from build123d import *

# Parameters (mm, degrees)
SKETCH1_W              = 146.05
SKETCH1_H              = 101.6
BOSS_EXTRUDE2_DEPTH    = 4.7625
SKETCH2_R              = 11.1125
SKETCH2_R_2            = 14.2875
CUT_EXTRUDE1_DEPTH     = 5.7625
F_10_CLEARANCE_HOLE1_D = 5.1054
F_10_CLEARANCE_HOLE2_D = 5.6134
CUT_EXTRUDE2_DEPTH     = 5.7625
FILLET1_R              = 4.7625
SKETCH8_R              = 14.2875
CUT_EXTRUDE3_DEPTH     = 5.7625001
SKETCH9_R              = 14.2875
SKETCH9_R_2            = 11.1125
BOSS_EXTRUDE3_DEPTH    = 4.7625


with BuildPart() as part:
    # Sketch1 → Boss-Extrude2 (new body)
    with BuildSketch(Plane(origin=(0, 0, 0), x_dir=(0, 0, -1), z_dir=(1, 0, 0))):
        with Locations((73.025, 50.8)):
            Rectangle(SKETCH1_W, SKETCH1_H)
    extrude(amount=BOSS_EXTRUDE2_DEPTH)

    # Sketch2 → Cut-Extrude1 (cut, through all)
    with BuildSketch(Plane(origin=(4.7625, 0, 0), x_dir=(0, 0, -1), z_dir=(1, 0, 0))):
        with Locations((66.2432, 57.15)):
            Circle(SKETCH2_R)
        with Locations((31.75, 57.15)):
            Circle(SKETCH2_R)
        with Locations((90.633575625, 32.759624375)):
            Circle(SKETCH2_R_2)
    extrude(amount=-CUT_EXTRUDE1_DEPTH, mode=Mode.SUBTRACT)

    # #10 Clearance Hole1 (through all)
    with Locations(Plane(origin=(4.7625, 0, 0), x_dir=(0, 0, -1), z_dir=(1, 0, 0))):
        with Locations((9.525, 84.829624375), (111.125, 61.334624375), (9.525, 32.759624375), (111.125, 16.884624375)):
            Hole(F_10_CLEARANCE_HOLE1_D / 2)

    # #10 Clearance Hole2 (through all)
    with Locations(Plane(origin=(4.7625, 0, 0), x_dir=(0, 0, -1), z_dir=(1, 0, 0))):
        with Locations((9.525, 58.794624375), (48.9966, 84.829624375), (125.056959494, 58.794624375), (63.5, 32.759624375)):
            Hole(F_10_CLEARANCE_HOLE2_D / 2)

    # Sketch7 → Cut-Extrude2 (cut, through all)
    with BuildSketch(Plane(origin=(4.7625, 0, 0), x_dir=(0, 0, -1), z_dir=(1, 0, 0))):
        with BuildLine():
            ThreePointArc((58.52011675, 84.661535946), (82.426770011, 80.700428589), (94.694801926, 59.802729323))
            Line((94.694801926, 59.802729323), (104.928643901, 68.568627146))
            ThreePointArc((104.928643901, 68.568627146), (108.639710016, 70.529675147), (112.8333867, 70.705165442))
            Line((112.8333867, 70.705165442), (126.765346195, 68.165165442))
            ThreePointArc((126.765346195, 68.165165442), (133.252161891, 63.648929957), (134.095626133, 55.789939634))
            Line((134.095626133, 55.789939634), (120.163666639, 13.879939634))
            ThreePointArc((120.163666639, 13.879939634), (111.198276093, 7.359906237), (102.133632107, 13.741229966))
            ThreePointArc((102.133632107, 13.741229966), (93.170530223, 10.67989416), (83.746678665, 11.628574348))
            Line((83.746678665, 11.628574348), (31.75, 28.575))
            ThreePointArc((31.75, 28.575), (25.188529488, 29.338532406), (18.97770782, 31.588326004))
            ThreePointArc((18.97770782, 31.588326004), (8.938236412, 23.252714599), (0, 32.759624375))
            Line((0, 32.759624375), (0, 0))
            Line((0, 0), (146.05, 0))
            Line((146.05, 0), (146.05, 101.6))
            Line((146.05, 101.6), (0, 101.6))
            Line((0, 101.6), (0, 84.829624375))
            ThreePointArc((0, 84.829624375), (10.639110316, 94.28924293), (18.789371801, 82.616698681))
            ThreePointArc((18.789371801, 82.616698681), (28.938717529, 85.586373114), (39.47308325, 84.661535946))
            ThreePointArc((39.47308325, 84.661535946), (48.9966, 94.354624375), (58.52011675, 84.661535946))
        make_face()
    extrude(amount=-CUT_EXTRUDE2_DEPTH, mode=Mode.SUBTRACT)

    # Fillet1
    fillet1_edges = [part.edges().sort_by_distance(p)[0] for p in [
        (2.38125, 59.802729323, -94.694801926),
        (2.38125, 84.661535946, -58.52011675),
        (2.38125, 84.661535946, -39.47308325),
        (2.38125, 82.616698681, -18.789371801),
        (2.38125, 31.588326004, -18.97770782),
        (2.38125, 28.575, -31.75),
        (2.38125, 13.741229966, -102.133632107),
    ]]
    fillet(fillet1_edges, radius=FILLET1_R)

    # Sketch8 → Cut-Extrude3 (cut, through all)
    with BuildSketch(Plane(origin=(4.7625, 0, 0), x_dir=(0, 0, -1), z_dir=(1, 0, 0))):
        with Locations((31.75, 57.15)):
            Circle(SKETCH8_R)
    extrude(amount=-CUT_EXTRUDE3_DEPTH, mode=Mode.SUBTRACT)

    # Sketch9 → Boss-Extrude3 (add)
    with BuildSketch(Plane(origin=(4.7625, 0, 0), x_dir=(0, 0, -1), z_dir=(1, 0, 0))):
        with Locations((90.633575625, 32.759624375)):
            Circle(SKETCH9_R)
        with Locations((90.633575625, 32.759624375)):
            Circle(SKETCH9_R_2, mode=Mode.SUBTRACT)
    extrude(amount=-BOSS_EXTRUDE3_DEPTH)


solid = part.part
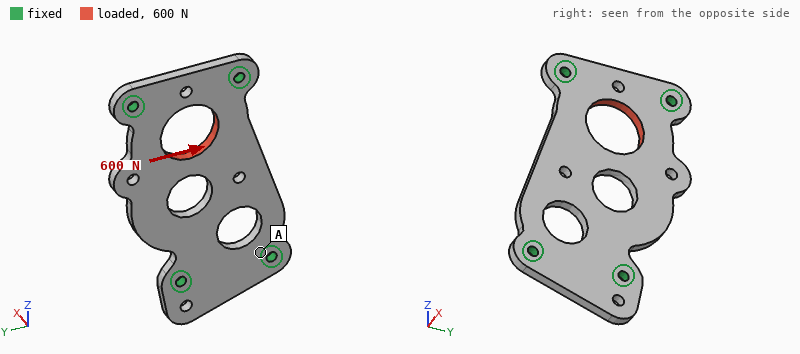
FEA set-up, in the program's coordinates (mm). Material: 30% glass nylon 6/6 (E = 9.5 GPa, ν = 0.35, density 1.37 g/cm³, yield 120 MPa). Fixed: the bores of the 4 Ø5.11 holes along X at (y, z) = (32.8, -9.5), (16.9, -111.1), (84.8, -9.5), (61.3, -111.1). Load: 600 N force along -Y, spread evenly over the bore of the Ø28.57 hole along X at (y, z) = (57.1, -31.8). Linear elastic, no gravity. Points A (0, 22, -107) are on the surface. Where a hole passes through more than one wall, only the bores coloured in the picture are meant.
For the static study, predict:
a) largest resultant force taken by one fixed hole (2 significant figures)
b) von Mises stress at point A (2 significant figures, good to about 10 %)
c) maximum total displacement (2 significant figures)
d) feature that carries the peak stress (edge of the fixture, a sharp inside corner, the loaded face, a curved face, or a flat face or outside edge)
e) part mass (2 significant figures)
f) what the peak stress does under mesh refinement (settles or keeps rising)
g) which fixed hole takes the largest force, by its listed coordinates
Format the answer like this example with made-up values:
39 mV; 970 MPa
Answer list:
260 N; 0.94 MPa; 29 µm; edge of the fixture; 43 g; keeps rising; (32.8, -9.5)
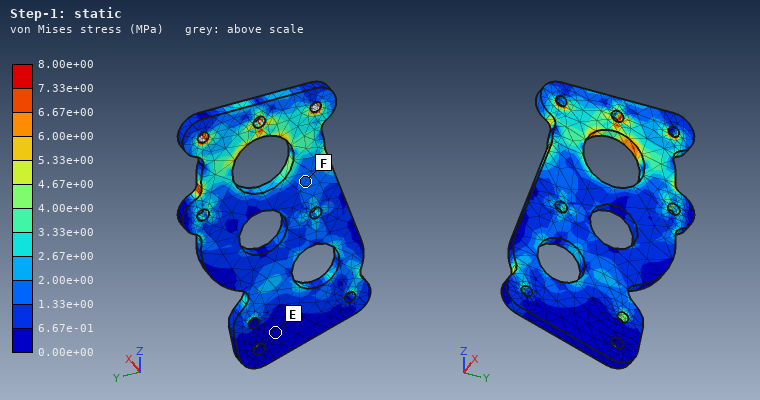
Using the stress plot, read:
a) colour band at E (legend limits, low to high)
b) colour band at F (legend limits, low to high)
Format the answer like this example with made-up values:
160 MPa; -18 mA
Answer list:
0.00e+00 to 6.67e-01 MPa; 1.33e+00 to 2.00e+00 MPa
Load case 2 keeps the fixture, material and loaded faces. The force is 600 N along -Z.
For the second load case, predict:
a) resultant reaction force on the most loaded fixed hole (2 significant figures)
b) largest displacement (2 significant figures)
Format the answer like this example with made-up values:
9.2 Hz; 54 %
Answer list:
240 N; 15 µm
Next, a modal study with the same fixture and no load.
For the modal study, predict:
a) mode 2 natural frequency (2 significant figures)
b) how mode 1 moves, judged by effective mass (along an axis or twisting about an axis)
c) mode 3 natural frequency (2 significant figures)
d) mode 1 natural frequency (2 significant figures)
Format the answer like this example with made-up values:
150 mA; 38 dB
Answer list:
1400 Hz; along X; 2900 Hz; 1100 Hz
